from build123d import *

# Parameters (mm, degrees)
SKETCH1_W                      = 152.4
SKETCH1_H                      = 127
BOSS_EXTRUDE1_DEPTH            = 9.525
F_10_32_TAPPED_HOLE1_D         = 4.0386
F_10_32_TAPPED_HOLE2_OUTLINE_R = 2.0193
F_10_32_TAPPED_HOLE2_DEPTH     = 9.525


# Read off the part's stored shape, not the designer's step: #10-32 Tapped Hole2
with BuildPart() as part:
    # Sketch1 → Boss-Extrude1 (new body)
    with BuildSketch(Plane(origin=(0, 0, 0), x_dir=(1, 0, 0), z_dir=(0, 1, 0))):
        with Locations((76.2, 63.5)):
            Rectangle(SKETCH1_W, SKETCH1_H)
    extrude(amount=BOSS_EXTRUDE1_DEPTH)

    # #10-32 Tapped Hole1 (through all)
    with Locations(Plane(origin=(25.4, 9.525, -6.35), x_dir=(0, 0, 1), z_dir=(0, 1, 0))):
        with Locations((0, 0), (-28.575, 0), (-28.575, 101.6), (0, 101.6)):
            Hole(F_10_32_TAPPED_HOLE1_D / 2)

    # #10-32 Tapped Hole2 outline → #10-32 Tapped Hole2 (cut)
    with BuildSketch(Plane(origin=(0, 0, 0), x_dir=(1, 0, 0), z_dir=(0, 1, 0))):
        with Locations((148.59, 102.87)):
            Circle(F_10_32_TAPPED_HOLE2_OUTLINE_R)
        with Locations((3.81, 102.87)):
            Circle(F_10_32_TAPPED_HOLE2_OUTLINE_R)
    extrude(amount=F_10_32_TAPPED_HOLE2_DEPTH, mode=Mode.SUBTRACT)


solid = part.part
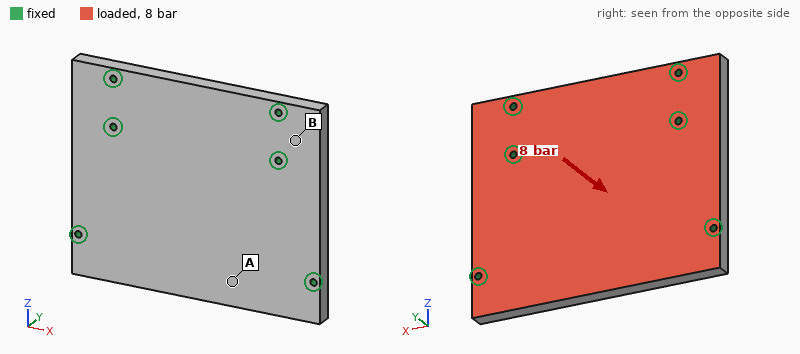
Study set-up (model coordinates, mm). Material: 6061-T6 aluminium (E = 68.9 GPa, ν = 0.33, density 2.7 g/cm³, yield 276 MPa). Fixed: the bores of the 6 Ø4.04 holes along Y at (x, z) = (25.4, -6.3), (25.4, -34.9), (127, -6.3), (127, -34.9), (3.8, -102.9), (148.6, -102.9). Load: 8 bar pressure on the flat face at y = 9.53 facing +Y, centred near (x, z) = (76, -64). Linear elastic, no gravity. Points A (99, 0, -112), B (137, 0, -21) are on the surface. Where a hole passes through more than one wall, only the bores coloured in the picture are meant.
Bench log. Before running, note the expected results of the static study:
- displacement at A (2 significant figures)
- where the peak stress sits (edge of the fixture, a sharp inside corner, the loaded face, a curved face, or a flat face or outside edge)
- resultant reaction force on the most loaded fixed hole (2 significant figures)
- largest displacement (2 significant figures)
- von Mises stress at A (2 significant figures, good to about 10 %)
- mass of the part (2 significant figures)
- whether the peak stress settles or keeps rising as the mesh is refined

0.23 mm
edge of the fixture
3.9 kN
0.31 mm
41 MPa
500 g
keeps rising
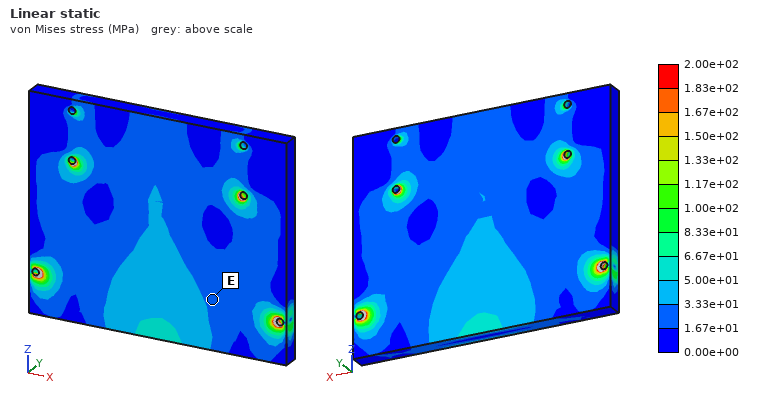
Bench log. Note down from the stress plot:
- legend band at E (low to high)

1.67e+01 to 3.33e+01 MPa
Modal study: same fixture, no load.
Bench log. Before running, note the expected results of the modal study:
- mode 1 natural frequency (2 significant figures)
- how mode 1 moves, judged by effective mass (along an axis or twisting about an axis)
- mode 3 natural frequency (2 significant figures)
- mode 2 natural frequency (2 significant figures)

2100 Hz
along Y
5400 Hz
4100 Hz
